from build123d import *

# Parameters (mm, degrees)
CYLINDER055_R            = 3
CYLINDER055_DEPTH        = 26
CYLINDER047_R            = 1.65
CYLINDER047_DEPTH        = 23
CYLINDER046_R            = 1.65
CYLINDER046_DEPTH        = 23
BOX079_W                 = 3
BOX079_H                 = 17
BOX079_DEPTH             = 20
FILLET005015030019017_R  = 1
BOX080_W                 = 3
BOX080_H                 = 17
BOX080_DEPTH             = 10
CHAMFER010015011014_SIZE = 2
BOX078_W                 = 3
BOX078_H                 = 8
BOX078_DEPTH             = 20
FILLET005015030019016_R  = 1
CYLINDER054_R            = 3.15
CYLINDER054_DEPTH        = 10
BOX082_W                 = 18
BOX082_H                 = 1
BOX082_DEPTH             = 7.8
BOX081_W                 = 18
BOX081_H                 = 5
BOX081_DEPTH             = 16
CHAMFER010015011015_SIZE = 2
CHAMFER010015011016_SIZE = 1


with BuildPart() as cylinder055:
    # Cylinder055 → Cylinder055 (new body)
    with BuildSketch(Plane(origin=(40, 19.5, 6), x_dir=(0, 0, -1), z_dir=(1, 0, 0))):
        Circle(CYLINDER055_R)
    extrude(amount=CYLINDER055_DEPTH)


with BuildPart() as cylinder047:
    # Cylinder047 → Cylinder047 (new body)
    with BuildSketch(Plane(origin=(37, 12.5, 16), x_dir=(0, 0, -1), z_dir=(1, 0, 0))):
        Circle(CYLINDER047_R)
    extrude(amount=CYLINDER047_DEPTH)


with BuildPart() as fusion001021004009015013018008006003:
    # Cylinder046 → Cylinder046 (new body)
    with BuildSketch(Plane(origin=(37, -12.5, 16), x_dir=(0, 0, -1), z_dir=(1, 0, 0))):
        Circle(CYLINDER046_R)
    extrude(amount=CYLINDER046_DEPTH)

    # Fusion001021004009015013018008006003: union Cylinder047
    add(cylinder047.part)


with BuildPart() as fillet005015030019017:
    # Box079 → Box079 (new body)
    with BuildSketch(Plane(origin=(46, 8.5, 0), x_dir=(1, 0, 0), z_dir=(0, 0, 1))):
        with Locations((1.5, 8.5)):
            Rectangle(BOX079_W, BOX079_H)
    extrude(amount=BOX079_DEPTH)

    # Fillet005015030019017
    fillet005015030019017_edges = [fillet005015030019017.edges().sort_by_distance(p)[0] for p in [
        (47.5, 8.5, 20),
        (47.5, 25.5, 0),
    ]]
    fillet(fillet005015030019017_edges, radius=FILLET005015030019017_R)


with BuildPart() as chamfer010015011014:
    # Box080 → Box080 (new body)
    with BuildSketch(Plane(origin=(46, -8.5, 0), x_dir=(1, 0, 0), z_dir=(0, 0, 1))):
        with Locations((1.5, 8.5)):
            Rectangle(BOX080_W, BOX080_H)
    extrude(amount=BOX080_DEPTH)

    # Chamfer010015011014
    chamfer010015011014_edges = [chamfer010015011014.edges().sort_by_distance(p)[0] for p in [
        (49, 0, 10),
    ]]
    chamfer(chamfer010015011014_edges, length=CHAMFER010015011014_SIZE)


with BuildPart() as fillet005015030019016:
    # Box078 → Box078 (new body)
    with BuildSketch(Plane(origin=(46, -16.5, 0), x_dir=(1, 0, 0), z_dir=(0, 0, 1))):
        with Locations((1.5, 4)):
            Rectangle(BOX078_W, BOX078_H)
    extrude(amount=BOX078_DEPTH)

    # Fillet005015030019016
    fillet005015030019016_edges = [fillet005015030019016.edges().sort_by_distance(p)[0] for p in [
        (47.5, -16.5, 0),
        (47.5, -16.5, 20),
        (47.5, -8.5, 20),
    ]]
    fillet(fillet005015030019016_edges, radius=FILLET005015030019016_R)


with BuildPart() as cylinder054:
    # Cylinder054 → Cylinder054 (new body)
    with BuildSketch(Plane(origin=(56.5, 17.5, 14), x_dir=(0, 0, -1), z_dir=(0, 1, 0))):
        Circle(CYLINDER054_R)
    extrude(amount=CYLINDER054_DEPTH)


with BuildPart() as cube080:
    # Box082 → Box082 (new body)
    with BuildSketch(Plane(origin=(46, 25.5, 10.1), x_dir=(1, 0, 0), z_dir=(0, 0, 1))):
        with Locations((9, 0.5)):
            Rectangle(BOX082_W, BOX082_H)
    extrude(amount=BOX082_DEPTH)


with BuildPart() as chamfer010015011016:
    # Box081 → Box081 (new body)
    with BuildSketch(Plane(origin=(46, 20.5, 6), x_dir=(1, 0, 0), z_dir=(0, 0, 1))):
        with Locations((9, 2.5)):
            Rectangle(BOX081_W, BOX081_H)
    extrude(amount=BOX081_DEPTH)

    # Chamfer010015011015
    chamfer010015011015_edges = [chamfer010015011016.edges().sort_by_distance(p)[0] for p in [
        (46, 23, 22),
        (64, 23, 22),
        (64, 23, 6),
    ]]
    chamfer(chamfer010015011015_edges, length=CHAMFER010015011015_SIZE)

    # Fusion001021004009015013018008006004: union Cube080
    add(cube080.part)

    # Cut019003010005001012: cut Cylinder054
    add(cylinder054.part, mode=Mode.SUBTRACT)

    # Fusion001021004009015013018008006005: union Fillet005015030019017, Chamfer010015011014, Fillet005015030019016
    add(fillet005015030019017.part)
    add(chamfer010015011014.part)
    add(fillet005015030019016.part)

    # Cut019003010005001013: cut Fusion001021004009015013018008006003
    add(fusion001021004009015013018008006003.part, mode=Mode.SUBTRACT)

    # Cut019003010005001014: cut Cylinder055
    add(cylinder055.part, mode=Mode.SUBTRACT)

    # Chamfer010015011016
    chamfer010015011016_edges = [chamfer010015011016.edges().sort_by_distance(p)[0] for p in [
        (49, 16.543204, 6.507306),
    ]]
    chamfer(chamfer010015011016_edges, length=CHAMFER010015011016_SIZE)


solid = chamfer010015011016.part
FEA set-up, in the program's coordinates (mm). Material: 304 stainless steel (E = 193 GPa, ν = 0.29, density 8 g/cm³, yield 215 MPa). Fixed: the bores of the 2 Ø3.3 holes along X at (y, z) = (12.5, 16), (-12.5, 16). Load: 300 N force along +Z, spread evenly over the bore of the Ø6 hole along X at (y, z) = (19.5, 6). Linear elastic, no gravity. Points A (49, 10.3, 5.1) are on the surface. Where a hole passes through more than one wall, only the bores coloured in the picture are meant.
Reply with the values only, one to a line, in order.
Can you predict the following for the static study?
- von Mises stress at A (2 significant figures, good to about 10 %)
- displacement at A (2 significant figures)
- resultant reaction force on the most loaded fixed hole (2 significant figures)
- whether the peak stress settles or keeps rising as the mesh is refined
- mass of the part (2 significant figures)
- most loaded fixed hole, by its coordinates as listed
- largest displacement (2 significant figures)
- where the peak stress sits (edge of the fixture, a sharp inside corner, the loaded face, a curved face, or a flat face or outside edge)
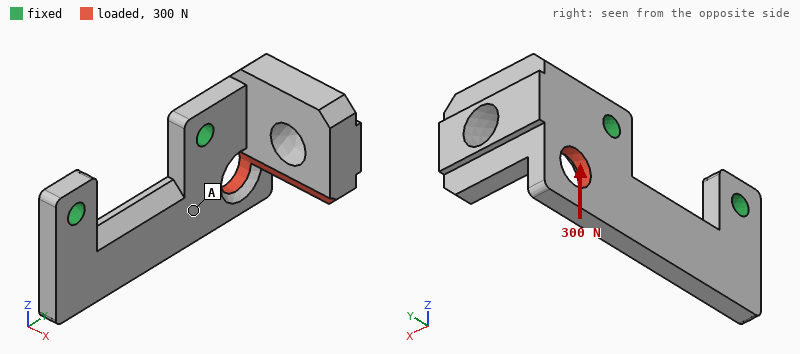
13 MPa
4.9 µm
350 N
keeps rising
23 g
(12.5, 16)
26 µm
edge of the fixture
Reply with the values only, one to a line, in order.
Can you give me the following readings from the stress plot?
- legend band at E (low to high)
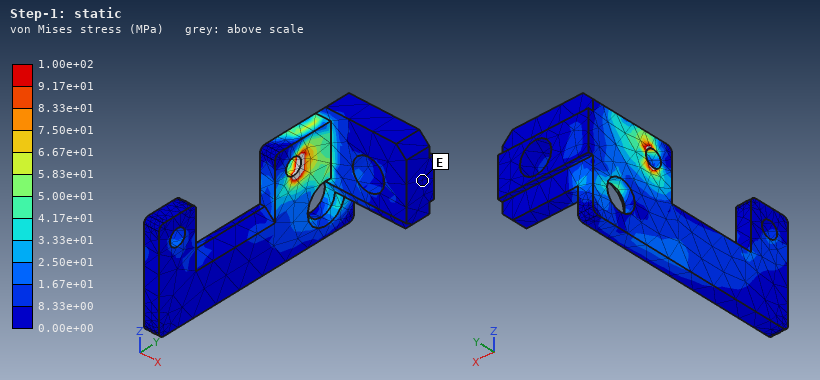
0.00e+00 to 8.33e+00 MPa
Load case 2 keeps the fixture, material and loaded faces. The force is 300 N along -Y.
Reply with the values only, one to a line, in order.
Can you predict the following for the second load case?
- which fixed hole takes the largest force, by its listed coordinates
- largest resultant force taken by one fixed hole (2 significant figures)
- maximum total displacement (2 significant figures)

(12.5, 16)
210 N
46 µm
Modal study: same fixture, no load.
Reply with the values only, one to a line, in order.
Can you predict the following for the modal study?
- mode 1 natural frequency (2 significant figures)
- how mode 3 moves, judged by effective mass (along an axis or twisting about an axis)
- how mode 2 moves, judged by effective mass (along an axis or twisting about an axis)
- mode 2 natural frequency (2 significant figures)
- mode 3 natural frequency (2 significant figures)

3500 Hz
along X
along Z
4600 Hz
7800 Hz
